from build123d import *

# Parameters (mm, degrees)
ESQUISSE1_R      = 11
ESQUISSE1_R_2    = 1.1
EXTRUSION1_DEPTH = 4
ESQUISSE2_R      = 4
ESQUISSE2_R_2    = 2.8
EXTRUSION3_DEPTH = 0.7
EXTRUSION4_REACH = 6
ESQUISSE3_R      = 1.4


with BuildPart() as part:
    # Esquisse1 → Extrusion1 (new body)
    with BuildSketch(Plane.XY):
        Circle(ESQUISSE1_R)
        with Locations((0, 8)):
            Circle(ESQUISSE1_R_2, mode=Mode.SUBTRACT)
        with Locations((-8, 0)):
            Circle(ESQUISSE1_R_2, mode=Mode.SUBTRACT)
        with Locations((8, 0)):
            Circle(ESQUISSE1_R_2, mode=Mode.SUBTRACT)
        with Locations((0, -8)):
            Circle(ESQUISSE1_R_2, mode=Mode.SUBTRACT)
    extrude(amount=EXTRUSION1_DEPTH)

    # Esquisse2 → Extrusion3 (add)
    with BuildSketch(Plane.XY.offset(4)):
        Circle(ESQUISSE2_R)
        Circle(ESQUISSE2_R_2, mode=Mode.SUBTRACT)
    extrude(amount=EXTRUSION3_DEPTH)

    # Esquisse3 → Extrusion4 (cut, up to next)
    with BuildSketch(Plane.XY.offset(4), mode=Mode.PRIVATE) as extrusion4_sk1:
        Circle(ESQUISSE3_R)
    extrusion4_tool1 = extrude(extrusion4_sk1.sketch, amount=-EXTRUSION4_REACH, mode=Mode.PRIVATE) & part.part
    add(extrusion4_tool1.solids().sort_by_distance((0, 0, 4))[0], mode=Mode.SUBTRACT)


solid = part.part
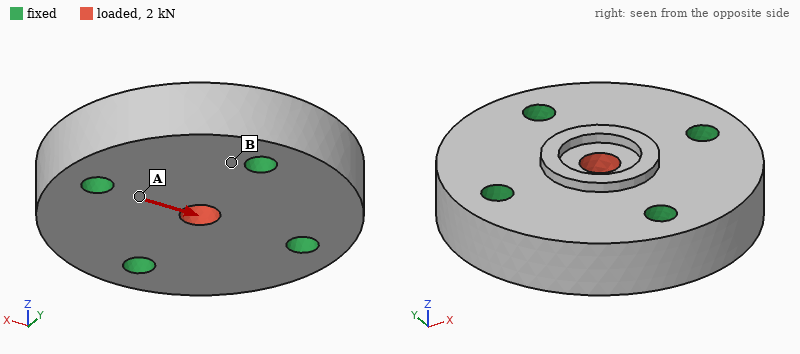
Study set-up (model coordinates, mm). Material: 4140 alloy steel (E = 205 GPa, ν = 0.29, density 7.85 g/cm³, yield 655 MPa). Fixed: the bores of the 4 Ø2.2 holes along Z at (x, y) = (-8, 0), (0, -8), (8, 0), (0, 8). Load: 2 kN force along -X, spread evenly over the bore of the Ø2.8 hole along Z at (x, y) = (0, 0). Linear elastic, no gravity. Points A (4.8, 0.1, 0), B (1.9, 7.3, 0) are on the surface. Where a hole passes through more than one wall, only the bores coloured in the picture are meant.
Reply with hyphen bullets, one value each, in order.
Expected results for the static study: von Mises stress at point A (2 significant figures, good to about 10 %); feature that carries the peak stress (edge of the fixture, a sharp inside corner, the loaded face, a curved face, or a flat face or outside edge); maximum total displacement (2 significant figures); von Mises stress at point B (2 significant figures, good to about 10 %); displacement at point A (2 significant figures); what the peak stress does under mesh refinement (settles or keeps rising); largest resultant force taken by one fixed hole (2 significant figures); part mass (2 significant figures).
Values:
- 45 MPa
- a sharp inside corner
- 1.3 µm
- 14 MPa
- 0.48 µm
- keeps rising
- 670 N
- 11 g
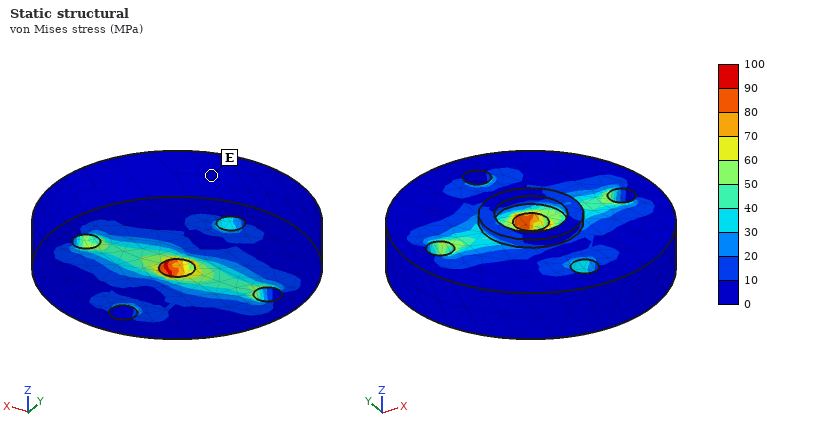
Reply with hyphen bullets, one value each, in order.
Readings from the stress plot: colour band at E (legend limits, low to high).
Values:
- 0 to 10 MPa
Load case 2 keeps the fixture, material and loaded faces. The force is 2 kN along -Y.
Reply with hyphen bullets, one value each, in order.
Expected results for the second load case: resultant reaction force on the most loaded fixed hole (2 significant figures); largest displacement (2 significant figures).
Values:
- 670 N
- 1.3 µm
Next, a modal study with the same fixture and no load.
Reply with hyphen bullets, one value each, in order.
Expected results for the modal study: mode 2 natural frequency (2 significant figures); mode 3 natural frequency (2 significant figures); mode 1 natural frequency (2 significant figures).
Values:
- 83 kHz
- 83 kHz
- 80 kHz
